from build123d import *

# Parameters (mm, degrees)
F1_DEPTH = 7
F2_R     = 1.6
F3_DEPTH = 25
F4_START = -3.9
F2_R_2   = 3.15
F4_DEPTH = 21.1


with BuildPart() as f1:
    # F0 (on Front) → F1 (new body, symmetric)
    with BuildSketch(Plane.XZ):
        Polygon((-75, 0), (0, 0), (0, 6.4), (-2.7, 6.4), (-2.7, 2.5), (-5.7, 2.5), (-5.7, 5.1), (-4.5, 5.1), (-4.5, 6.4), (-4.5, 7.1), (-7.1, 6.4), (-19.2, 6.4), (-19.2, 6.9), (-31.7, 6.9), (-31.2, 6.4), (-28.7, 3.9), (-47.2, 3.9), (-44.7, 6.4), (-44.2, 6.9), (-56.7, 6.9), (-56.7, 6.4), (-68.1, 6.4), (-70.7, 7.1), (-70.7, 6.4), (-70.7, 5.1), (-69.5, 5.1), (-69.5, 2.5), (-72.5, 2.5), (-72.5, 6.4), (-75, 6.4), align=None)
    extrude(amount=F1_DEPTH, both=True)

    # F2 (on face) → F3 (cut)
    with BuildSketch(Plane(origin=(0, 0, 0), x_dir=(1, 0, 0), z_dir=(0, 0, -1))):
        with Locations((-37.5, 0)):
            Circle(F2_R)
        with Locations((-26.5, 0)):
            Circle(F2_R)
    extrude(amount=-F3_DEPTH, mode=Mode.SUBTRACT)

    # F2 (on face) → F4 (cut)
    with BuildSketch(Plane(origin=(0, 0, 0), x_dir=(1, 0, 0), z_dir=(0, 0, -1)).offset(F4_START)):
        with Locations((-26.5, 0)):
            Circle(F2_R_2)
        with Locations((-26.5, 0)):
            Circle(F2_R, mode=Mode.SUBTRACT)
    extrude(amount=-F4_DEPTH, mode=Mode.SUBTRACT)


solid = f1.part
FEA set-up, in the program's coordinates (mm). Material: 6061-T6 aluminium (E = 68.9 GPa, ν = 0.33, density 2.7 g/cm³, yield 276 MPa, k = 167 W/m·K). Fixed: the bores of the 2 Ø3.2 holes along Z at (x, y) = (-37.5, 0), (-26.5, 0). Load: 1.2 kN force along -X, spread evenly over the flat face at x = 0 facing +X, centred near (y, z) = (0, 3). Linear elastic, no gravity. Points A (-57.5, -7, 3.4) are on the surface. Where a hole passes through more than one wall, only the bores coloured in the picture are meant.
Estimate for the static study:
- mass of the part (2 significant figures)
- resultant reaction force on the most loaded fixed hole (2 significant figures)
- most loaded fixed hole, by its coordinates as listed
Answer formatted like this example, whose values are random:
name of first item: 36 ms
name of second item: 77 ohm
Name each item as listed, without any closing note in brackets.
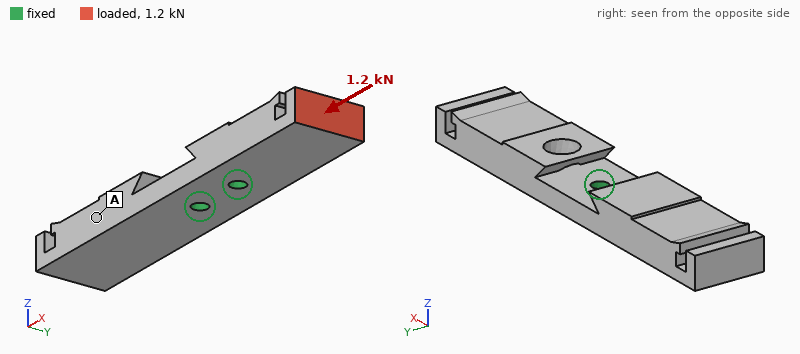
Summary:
mass of the part: 16 g
resultant reaction force on the most loaded fixed hole: 970 N
most loaded fixed hole, by its coordinates as listed: (-26.5, 0)
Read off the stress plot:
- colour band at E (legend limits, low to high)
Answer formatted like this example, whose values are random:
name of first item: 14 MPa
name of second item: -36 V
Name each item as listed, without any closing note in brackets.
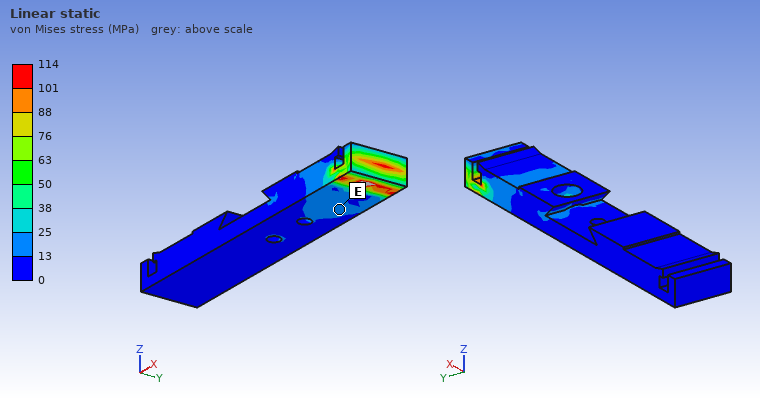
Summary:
colour band at E: 13 to 25 MPa
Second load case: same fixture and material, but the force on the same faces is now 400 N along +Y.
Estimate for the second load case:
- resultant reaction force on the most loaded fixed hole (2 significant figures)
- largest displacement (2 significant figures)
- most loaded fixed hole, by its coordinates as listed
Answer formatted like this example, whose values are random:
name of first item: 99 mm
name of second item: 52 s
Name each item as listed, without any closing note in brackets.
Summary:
resultant reaction force on the most loaded fixed hole: 1.0 kN
largest displacement: 68 µm
most loaded fixed hole, by its coordinates as listed: (-26.5, 0)
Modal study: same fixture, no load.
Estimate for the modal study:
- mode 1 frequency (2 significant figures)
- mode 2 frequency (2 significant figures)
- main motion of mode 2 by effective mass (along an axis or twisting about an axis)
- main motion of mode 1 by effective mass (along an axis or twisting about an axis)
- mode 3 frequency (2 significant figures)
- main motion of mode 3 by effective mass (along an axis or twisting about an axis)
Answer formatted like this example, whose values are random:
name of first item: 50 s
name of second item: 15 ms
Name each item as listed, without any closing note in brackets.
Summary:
mode 1 frequency: 2100 Hz
mode 2 frequency: 5100 Hz
main motion of mode 2 by effective mass: along Y
main motion of mode 1 by effective mass: along Z
mode 3 frequency: 5800 Hz
main motion of mode 3 by effective mass: along Z
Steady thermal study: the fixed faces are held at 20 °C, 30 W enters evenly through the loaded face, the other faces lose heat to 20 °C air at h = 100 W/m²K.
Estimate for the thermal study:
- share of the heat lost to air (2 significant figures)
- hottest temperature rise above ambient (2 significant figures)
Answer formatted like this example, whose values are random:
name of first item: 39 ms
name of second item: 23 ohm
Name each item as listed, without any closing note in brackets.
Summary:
share of the heat lost to air: 14 %
hottest temperature rise above ambient: 73 K
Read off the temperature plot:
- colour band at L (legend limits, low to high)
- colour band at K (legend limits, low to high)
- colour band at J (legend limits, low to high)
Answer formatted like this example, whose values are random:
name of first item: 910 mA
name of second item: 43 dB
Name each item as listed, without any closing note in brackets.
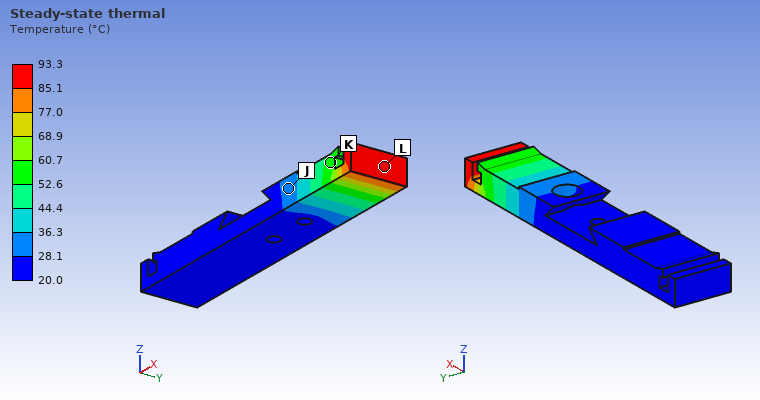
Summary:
colour band at L: 85.1 to 93.3 °C
colour band at K: 52.6 to 60.7 °C
colour band at J: 28.1 to 36.3 °C
